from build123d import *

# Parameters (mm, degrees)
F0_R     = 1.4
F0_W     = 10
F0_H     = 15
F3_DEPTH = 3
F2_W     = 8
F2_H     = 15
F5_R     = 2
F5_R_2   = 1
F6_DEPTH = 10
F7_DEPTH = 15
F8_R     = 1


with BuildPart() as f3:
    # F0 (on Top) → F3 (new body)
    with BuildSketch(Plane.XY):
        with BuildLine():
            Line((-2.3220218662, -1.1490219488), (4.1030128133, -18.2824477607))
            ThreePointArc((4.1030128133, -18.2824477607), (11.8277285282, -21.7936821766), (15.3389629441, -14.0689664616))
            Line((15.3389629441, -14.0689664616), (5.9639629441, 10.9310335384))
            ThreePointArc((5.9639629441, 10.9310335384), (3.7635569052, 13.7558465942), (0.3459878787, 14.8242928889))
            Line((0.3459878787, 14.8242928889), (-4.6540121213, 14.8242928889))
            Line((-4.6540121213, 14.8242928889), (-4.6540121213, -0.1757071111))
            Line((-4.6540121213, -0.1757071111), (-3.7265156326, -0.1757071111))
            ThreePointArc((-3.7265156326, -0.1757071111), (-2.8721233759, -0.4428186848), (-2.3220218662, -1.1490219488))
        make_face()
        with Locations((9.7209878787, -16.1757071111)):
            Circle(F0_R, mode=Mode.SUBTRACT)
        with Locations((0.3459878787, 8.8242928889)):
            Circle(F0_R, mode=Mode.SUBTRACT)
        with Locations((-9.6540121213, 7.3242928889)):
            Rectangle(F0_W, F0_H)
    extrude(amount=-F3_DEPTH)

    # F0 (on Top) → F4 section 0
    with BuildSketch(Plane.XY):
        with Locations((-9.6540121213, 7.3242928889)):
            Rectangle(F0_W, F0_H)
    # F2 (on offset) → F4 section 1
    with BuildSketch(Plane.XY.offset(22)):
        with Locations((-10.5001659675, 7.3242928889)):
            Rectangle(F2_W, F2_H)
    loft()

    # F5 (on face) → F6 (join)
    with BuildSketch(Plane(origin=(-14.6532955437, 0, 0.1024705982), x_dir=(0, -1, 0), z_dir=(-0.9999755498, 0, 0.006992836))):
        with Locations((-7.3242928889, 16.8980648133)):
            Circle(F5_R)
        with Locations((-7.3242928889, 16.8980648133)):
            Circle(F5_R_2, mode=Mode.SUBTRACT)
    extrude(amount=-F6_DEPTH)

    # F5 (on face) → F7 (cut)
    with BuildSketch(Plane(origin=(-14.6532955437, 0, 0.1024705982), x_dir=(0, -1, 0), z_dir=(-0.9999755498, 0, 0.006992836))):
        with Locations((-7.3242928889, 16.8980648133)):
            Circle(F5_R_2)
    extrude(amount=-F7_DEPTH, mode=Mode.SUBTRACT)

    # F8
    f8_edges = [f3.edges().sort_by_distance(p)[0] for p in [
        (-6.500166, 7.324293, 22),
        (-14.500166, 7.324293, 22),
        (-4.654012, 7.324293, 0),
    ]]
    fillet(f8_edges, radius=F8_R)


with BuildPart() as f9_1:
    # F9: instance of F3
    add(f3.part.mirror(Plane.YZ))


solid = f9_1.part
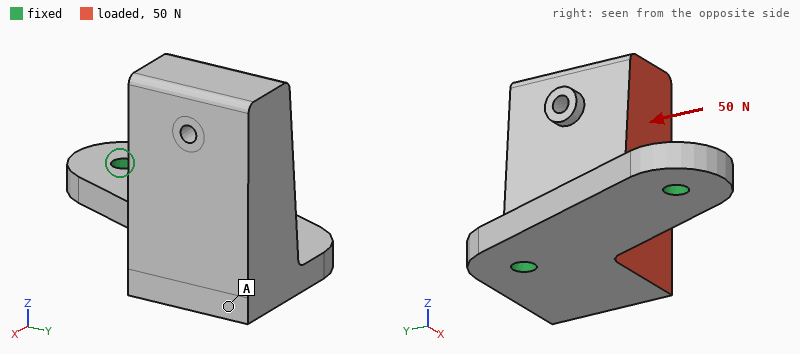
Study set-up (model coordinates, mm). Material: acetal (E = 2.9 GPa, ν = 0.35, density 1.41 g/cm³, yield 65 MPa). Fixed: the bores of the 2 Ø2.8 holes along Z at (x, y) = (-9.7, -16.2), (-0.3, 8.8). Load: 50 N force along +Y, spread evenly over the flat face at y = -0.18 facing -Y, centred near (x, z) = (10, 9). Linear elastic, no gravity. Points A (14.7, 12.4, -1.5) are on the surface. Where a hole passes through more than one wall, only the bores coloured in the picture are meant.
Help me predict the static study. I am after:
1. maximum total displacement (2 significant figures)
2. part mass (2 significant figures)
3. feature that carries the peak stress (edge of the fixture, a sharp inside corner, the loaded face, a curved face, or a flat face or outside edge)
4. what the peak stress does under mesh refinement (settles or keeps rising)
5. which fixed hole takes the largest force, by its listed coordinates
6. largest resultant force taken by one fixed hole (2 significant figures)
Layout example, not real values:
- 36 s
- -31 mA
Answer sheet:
- 0.41 mm
- 6.6 g
- edge of the fixture
- keeps rising
- (-0.3, 8.8)
- 48 N
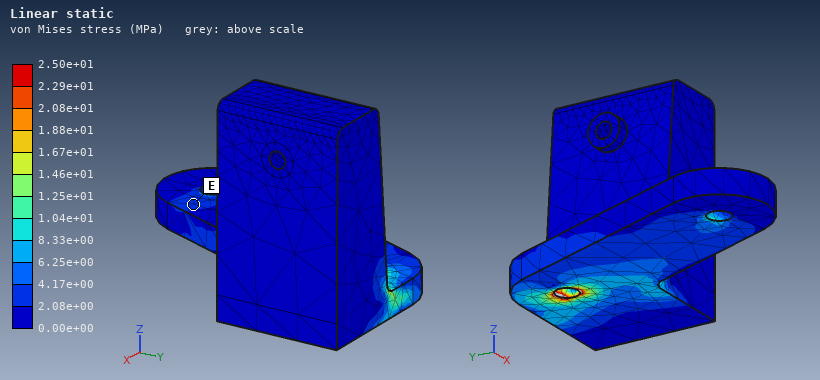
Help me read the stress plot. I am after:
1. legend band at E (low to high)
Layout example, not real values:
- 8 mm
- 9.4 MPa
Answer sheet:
- 2.08e+00 to 4.17e+00 MPa
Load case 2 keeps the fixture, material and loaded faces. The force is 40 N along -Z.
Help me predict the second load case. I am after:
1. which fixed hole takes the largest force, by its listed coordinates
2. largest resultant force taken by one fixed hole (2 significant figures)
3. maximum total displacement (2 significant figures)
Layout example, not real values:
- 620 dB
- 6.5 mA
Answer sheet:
- (-0.3, 8.8)
- 38 N
- 0.62 mm
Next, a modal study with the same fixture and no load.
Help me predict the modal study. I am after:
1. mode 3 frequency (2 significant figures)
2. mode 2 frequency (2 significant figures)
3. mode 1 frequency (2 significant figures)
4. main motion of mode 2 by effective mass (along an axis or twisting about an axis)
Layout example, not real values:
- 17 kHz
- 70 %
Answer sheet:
- 3600 Hz
- 980 Hz
- 610 Hz
- along Y
